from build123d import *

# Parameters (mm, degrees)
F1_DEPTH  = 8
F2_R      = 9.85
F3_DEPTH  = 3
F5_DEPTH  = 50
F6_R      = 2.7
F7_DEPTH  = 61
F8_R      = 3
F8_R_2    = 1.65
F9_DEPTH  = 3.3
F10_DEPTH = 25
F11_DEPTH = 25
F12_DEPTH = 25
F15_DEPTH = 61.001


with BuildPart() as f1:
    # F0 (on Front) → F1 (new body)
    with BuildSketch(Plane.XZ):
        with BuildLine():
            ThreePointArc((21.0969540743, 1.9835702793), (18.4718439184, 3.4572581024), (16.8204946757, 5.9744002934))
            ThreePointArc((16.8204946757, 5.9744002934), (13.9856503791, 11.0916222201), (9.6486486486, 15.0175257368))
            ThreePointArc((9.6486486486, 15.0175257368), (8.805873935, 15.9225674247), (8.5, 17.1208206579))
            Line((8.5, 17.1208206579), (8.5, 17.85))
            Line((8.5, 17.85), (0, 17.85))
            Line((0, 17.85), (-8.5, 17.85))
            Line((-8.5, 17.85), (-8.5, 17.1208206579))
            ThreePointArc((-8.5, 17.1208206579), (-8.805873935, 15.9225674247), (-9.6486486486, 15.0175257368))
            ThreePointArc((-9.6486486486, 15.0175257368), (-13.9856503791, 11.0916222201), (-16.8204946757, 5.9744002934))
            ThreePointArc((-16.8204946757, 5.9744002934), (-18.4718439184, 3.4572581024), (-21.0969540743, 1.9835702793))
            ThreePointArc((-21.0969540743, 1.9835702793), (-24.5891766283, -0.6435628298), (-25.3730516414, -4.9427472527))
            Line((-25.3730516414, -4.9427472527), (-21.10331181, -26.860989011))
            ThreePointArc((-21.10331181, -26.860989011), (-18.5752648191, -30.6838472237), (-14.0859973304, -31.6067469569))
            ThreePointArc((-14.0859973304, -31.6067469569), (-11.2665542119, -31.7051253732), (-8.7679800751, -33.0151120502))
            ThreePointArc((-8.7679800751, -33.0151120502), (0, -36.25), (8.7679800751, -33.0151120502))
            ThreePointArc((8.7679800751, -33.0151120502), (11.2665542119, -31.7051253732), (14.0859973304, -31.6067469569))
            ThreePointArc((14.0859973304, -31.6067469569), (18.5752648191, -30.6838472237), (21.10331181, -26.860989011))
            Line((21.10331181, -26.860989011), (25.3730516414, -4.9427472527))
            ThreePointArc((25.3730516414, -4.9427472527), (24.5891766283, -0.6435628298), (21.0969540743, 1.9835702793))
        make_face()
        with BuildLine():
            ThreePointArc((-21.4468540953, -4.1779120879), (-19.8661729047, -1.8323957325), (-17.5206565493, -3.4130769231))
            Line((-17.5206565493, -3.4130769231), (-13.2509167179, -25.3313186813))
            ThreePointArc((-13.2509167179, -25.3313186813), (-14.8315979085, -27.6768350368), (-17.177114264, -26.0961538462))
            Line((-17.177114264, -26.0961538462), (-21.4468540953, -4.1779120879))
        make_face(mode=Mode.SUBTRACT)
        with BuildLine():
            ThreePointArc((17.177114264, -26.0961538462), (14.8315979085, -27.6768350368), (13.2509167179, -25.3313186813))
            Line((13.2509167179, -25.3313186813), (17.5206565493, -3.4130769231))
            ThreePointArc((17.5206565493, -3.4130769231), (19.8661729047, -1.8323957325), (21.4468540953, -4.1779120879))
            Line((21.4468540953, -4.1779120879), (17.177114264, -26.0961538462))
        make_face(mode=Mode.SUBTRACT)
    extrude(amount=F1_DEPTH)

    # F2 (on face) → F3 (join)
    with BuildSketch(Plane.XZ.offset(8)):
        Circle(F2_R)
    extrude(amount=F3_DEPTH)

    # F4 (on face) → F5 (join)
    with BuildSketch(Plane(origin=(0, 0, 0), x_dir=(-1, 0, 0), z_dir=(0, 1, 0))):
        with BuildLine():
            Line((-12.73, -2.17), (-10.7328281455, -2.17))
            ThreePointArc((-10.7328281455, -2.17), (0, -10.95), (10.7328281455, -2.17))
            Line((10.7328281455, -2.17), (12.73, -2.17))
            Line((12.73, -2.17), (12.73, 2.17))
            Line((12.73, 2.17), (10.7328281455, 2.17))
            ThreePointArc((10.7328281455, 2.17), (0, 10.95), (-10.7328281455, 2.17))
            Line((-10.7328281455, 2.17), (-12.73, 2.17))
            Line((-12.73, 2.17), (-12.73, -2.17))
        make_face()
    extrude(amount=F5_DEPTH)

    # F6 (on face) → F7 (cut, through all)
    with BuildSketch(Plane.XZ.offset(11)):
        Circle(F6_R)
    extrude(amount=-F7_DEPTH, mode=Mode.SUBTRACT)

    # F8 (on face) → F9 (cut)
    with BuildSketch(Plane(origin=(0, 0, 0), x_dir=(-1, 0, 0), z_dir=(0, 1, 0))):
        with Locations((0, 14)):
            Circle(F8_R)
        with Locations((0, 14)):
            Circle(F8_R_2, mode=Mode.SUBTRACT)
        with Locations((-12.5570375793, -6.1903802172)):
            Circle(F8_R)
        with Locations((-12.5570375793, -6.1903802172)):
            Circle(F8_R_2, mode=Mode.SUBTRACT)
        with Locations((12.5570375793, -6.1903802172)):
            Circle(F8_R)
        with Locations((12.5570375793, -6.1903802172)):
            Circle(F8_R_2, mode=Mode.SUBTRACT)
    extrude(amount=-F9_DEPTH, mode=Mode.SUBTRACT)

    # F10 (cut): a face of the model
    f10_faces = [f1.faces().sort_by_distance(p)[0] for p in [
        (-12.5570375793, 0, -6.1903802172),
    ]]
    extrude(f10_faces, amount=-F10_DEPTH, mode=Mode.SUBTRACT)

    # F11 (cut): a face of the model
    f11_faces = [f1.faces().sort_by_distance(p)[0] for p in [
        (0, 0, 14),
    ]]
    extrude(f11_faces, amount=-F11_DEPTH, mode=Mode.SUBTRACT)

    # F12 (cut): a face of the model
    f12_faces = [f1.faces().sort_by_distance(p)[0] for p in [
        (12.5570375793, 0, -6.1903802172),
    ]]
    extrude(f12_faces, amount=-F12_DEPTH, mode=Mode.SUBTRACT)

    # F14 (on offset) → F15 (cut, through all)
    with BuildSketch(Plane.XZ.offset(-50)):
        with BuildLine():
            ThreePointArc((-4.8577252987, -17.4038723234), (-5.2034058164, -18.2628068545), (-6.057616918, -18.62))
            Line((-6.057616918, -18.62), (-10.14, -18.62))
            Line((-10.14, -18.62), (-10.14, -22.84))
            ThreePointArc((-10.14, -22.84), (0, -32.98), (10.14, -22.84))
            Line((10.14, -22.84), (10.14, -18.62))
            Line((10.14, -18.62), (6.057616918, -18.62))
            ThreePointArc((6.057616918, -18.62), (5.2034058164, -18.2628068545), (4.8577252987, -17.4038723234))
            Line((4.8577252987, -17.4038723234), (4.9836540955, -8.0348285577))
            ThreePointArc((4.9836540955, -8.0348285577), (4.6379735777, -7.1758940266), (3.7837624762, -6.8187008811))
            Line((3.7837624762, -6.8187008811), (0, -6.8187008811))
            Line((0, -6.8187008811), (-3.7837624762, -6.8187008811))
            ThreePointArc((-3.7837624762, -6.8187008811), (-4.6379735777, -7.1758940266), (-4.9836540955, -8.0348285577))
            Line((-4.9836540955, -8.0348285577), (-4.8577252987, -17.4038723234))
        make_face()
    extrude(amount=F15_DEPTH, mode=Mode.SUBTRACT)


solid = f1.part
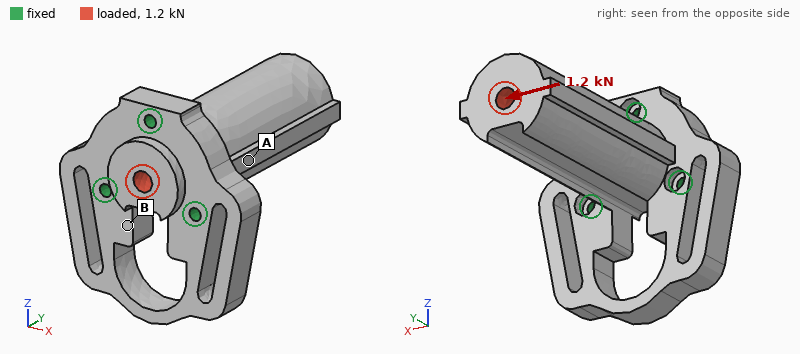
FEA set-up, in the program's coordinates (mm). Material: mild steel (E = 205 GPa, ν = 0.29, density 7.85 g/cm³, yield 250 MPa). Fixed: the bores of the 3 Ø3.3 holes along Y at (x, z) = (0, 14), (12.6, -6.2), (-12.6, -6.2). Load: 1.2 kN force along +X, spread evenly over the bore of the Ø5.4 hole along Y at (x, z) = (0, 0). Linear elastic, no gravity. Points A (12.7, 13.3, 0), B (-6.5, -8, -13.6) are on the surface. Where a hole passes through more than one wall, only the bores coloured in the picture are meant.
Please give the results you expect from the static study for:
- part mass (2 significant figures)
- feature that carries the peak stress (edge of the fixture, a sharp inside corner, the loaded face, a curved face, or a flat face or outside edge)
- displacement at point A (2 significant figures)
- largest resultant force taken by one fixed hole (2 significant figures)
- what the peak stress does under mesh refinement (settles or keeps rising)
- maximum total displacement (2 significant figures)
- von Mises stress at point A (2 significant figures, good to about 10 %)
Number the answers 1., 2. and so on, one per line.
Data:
1. 230 g
2. edge of the fixture
3. 5.0 µm
4. 1.3 kN
5. keeps rising
6. 15 µm
7. 12 MPa
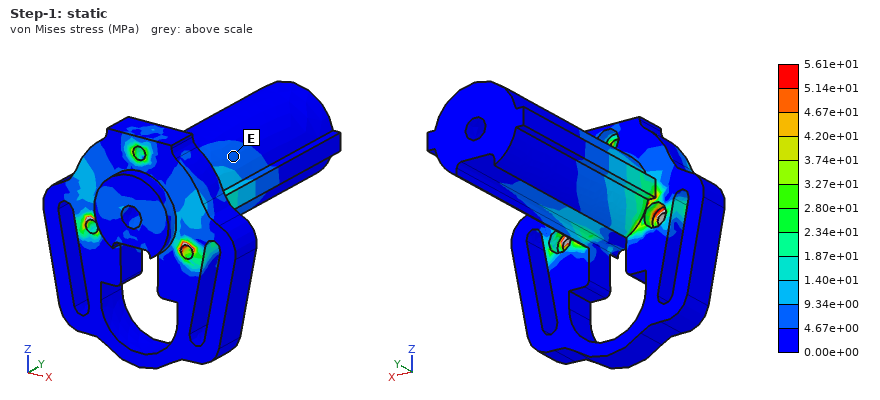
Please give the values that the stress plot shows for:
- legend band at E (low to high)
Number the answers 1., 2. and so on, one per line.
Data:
1. 4.67e+00 to 9.34e+00 MPa
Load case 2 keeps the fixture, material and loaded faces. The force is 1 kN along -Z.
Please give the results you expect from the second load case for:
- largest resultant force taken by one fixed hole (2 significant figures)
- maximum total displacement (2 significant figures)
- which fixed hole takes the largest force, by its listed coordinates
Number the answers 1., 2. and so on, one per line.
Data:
1. 1.3 kN
2. 17 µm
3. (0, 14)
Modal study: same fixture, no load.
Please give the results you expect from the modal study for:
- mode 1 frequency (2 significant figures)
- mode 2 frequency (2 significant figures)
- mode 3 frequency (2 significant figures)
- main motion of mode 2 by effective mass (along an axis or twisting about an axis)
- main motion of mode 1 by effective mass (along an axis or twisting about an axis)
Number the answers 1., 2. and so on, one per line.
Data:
1. 3700 Hz
2. 4300 Hz
3. 6500 Hz
4. along X
5. along Z
